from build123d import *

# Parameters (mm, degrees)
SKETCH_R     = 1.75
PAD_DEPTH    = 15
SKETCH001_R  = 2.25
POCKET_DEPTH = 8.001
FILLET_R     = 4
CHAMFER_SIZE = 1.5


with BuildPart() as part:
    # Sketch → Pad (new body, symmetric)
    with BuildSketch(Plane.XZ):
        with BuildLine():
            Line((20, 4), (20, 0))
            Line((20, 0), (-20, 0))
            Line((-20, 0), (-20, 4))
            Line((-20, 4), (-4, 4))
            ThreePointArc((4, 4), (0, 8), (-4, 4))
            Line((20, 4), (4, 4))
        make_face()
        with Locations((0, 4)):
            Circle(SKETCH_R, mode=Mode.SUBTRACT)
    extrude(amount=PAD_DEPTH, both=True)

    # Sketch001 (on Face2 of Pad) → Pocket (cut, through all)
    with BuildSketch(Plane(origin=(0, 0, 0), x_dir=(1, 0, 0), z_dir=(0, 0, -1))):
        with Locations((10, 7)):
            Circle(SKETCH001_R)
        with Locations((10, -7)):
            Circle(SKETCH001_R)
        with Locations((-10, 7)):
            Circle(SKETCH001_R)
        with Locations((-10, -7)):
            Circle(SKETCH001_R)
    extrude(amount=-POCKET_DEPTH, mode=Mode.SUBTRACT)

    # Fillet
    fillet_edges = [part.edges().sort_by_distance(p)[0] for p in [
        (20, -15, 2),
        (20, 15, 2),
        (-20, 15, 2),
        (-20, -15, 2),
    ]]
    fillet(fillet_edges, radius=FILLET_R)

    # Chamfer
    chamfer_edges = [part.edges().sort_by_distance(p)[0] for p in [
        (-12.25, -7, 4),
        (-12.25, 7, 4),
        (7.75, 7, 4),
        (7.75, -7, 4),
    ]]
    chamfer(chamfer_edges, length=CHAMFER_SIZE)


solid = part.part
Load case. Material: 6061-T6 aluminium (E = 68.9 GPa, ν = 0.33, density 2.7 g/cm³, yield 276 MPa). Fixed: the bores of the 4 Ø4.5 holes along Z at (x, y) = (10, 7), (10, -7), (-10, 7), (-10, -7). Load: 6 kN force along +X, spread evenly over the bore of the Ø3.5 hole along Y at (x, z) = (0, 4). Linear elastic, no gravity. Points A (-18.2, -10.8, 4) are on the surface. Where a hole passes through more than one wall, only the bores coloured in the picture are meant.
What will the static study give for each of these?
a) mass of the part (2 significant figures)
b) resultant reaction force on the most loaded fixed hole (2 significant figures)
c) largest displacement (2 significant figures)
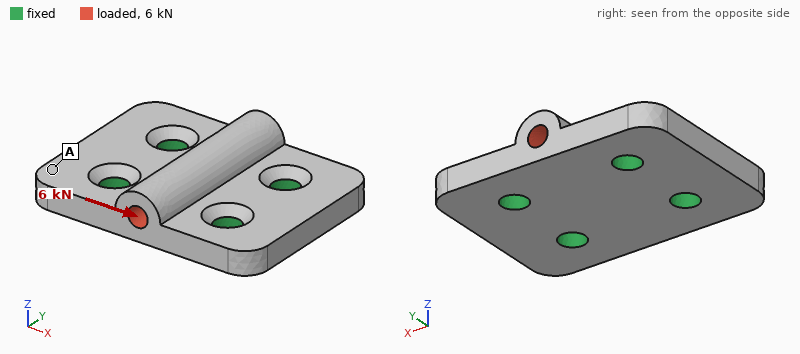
13 g
1.6 kN
7.7 µm
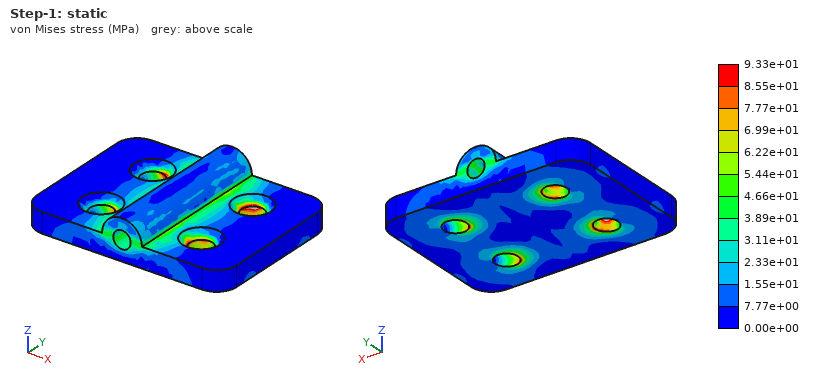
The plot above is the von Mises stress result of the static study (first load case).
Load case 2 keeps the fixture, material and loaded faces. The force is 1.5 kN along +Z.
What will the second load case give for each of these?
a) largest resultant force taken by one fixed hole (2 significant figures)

410 N
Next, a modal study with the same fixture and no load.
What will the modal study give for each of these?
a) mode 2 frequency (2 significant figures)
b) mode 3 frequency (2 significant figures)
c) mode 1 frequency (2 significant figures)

28 kHz
32 kHz
27 kHz
